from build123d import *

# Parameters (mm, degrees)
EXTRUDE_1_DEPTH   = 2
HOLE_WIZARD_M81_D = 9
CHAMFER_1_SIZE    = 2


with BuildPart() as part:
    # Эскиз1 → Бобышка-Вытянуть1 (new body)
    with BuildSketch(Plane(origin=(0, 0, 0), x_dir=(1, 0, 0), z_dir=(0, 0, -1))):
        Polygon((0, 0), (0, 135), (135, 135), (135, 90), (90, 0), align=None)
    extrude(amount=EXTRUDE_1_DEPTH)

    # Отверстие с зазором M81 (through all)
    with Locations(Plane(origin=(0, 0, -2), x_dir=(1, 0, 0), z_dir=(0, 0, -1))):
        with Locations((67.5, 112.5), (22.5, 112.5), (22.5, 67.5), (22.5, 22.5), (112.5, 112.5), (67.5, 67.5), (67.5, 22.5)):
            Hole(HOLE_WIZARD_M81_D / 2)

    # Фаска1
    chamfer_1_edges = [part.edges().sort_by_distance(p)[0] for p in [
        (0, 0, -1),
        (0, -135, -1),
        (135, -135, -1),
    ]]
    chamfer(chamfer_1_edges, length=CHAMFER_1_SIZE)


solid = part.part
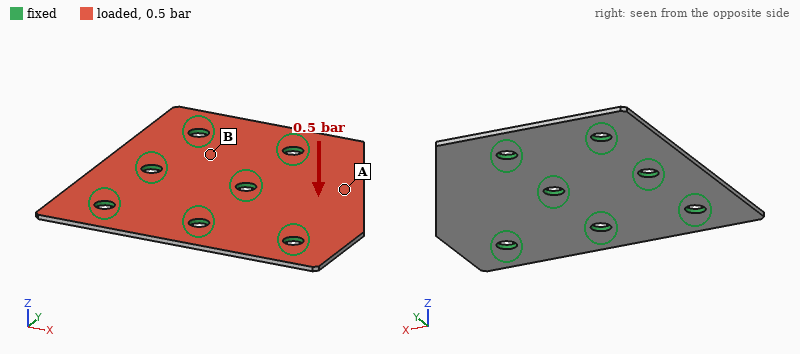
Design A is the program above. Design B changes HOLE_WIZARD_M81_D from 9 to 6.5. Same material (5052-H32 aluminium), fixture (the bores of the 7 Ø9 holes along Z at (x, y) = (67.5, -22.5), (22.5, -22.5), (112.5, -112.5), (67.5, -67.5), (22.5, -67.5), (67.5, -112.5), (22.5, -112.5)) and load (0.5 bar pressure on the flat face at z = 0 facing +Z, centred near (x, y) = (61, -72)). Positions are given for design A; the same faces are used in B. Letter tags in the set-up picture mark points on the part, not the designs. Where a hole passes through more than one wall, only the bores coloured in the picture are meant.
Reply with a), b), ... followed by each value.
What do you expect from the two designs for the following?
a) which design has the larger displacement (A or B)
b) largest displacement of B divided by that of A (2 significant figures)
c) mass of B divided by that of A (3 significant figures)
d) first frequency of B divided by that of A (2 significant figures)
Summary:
a) B
b) 1.1
c) 1.01
d) 0.94
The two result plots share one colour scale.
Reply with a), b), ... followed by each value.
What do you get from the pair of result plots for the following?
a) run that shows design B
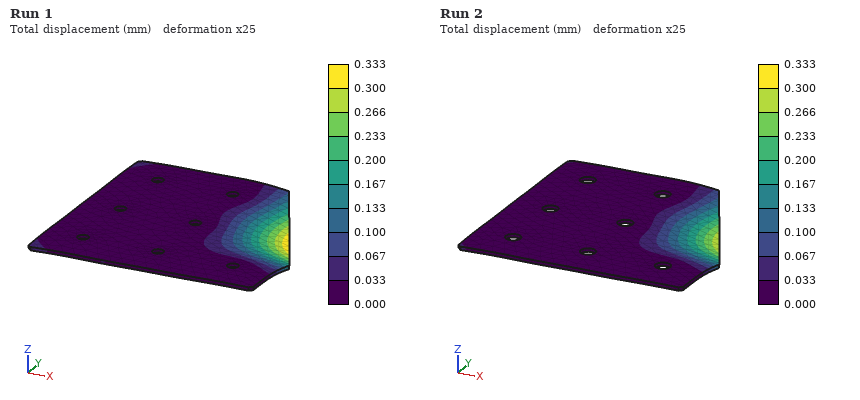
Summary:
a) Run 1
